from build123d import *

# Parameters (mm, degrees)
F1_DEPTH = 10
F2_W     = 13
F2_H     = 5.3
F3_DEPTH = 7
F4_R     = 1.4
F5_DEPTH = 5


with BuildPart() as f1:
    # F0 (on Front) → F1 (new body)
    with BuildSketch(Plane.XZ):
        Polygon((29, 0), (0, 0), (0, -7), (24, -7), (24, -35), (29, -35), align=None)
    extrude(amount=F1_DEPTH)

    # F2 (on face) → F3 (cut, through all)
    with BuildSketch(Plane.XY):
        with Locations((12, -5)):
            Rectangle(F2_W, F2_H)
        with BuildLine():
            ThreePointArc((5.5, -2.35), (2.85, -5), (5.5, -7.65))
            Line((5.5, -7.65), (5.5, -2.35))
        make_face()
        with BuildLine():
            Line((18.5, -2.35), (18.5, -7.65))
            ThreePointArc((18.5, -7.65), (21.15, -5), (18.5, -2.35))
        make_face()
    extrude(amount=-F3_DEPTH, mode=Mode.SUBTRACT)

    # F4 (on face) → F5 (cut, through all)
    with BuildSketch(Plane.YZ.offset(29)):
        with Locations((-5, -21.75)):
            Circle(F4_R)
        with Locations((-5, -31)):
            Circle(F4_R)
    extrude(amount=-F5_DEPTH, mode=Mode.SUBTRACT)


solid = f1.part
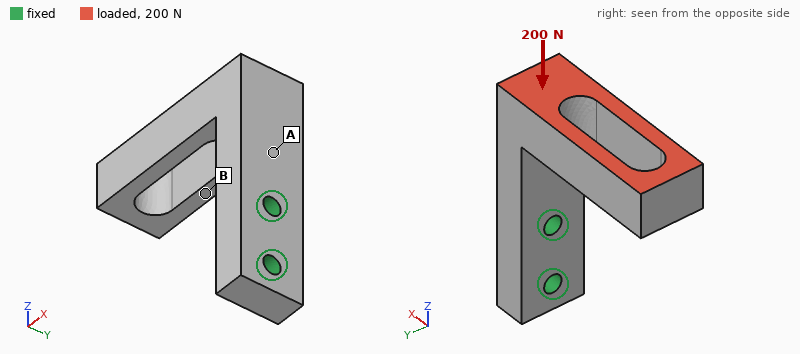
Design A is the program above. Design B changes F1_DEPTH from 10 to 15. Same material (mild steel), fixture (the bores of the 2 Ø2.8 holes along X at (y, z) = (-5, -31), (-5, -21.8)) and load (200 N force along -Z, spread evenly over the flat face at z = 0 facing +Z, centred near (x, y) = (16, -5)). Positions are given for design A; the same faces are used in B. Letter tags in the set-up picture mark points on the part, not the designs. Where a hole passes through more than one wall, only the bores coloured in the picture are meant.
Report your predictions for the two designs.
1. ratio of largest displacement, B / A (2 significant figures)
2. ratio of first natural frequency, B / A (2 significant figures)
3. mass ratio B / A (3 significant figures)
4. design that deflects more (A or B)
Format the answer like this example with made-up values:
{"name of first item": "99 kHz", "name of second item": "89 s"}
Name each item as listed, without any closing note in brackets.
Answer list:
{"ratio of largest displacement, B / A": "0.70", "ratio of first natural frequency, B / A": "0.90", "mass ratio B / A": "1.63", "design that deflects more": "A"}
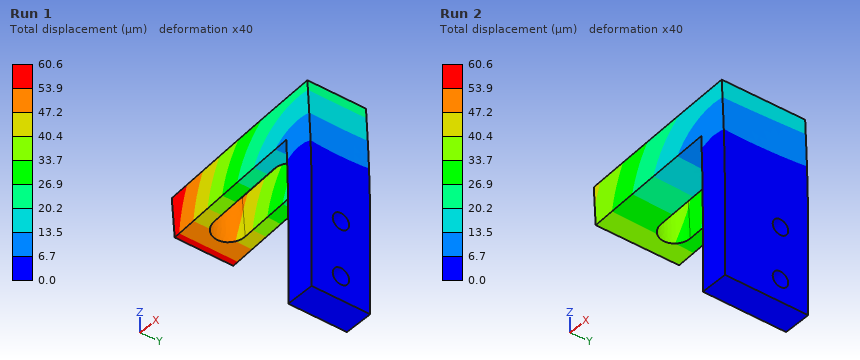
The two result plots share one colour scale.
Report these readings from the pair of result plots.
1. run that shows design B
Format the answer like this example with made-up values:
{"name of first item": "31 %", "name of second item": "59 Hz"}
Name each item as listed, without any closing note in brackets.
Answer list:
{"run that shows design B": "Run 2"}
